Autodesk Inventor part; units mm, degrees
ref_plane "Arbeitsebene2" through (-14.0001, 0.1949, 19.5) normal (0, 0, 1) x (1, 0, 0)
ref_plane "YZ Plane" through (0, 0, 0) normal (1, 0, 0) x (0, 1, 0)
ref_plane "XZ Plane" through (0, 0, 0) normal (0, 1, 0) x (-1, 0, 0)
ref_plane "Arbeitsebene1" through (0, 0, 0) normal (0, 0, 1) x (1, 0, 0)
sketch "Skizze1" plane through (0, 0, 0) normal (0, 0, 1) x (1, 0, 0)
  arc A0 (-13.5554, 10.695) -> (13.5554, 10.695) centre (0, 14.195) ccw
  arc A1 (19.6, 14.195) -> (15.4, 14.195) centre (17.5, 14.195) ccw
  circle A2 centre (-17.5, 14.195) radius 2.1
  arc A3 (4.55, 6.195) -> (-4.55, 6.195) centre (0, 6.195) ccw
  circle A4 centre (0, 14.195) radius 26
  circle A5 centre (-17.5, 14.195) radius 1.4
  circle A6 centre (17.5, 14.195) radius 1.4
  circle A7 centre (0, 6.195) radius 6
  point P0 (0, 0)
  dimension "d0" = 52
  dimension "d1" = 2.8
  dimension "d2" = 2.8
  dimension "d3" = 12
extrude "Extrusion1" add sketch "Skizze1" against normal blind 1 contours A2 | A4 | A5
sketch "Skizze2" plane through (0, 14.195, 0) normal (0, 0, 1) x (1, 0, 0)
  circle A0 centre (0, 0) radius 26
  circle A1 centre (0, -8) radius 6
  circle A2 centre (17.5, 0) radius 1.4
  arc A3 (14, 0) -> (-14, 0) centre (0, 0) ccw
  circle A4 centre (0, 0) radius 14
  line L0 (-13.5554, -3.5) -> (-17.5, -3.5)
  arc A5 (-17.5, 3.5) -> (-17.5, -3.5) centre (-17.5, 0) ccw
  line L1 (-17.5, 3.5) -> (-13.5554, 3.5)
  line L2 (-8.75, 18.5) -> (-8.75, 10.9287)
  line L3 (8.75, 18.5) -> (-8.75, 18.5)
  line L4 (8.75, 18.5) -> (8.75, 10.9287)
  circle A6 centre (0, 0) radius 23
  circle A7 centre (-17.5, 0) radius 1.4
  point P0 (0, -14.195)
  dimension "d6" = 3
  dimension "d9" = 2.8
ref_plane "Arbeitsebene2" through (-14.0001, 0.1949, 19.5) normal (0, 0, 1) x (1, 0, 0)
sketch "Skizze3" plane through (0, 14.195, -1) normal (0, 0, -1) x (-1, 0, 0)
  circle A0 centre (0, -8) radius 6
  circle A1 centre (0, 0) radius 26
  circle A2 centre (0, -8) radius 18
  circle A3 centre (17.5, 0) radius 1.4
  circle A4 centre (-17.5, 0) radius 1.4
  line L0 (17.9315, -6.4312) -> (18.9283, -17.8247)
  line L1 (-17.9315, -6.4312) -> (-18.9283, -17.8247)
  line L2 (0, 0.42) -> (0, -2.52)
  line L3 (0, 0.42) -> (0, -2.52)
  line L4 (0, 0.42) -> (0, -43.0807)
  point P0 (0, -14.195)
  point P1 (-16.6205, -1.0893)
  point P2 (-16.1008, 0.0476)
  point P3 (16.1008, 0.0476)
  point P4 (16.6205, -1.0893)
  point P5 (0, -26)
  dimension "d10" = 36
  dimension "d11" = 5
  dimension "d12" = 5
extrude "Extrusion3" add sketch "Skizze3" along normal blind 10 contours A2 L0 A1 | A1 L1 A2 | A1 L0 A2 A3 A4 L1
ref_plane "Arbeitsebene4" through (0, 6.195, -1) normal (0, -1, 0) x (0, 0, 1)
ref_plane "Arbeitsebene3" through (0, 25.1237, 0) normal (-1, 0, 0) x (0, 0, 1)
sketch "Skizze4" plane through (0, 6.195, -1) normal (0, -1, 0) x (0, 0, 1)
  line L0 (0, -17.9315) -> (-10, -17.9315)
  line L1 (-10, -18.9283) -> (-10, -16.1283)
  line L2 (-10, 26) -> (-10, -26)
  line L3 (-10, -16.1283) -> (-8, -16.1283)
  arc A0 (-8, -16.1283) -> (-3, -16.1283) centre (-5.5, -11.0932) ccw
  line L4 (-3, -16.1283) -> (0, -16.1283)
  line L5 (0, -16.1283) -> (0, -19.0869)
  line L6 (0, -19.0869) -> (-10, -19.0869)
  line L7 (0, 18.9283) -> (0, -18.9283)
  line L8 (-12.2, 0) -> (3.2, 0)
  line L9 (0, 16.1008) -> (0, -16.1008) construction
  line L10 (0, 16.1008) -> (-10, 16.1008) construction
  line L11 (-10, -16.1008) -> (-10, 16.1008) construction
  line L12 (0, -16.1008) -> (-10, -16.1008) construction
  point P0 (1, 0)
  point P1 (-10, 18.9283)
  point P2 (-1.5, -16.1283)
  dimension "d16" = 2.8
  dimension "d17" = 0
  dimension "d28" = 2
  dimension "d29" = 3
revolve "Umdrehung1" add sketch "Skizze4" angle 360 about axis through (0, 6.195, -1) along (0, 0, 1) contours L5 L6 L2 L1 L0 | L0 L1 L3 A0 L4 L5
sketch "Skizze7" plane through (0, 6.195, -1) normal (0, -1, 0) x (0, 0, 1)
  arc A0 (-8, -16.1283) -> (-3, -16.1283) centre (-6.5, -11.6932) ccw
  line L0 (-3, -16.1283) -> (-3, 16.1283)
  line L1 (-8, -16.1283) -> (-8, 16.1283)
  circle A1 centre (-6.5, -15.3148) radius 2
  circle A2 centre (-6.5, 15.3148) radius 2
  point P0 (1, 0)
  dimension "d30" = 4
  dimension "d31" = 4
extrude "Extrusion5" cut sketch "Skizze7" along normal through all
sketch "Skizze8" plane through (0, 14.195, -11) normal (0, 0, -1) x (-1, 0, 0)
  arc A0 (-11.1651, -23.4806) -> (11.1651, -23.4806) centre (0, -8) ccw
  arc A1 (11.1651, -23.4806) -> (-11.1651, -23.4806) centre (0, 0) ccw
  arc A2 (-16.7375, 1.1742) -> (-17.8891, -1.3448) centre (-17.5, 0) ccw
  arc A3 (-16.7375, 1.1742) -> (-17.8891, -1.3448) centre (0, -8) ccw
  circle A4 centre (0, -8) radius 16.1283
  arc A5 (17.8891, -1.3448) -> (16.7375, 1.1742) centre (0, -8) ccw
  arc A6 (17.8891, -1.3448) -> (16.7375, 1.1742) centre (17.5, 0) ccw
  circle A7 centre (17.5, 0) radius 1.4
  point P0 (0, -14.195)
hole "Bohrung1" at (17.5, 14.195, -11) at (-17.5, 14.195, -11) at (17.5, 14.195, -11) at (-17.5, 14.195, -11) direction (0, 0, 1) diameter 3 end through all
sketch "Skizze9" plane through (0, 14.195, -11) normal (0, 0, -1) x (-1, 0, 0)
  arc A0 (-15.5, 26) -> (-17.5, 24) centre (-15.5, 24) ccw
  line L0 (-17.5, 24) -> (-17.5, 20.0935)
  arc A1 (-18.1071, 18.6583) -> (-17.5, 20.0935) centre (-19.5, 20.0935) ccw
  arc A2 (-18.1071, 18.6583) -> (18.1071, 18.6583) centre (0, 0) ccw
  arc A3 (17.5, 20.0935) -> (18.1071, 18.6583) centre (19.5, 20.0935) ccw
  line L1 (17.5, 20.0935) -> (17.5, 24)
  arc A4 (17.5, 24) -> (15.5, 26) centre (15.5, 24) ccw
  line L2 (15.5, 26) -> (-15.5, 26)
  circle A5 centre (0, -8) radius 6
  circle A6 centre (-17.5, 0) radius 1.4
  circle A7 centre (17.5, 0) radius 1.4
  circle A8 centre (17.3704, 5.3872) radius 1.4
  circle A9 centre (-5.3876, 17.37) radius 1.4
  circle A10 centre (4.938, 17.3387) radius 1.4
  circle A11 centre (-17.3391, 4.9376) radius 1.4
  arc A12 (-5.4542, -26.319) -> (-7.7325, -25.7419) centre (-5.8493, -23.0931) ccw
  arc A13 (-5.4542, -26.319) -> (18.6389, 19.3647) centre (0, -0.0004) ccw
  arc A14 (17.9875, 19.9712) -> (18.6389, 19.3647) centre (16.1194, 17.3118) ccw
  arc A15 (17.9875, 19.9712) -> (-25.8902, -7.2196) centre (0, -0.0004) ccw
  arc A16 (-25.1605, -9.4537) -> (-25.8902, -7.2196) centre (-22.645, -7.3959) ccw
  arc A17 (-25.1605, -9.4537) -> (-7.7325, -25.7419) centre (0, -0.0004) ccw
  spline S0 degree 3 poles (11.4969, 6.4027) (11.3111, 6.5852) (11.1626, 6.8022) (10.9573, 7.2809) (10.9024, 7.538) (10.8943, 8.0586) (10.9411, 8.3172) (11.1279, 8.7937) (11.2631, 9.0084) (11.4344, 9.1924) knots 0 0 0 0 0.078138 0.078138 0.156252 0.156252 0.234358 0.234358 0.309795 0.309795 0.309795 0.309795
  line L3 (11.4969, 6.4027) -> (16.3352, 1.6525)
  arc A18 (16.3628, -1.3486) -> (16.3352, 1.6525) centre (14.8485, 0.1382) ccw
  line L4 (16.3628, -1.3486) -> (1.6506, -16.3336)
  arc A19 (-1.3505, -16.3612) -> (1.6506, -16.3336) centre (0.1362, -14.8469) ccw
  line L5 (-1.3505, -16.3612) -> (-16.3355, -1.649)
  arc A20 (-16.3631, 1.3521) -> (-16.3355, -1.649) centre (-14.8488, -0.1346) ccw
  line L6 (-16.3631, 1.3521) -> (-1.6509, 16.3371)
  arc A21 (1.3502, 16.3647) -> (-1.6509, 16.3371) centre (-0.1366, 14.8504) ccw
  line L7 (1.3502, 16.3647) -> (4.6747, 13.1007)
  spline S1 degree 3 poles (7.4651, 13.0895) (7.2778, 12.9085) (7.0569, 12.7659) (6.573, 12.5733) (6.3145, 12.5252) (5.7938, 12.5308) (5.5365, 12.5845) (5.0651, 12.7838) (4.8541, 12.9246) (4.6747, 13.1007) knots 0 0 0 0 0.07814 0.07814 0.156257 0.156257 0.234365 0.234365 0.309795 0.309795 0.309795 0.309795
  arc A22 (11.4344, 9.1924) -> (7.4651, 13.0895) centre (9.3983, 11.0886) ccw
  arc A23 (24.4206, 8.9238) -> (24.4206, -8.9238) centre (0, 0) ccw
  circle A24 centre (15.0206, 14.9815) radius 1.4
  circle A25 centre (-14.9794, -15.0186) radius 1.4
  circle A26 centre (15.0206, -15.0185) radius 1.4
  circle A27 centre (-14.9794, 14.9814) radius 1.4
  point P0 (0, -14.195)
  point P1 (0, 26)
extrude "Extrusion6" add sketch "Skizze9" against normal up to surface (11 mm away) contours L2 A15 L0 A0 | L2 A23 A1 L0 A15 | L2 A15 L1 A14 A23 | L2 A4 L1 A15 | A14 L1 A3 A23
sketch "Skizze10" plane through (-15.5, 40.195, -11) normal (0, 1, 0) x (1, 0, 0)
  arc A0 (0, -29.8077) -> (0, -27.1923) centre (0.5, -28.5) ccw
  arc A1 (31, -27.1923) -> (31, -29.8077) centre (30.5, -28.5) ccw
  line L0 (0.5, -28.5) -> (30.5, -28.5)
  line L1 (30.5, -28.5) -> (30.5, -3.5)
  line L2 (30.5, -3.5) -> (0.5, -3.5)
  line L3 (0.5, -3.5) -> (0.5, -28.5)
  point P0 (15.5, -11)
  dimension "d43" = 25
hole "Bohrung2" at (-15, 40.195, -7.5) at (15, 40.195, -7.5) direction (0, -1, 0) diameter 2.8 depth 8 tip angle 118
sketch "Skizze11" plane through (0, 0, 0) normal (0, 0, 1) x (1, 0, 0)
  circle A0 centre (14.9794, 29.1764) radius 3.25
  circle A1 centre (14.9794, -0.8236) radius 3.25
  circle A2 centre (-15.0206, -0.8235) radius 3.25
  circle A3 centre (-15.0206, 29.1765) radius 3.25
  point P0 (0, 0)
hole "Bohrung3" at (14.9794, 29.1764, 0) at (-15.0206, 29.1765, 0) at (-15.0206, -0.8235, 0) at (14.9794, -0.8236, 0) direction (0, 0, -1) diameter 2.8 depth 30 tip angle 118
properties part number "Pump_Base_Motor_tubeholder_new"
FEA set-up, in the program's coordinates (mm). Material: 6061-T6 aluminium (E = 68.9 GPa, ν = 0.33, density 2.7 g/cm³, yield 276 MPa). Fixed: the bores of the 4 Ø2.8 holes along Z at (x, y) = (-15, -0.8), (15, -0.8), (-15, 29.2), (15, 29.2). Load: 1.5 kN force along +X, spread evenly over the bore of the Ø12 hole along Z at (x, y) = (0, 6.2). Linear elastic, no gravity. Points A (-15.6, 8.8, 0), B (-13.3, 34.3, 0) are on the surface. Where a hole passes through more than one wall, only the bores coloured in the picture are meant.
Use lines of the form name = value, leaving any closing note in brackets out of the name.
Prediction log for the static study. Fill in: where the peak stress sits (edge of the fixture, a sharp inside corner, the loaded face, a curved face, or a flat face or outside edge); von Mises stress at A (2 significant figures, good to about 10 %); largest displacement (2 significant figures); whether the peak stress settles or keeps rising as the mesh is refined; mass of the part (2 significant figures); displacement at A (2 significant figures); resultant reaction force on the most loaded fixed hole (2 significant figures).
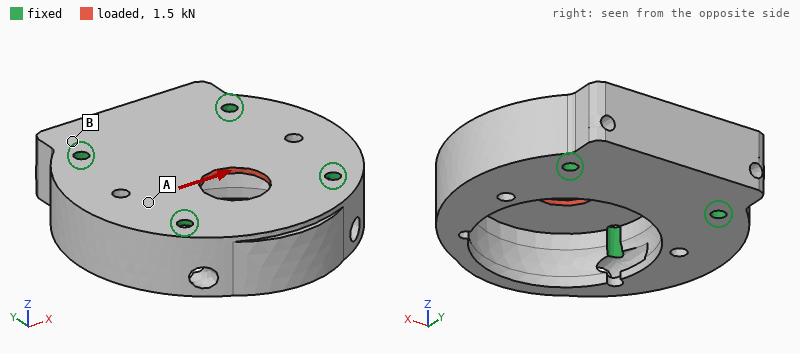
where the peak stress sits = edge of the fixture
von Mises stress at A = 18 MPa
largest displacement = 7.6 µm
whether the peak stress settles or keeps rising as the mesh is refined = keeps rising
mass of the part = 41 g
displacement at A = 3.3 µm
resultant reaction force on the most loaded fixed hole = 500 N
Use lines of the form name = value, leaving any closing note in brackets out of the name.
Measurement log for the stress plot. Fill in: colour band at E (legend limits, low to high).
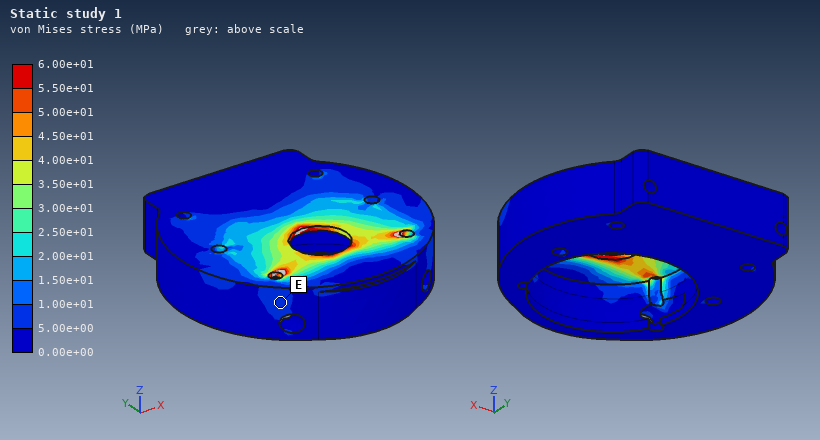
colour band at E = 5.00e+00 to 1.00e+01 MPa
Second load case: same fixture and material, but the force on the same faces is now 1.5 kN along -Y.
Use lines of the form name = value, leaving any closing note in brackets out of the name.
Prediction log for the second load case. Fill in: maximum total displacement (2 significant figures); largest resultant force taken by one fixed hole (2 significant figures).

maximum total displacement = 13 µm
largest resultant force taken by one fixed hole = 400 N
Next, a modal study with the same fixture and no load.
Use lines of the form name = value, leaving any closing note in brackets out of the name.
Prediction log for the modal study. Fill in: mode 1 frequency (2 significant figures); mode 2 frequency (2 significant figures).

mode 1 frequency = 12 kHz
mode 2 frequency = 17 kHz
